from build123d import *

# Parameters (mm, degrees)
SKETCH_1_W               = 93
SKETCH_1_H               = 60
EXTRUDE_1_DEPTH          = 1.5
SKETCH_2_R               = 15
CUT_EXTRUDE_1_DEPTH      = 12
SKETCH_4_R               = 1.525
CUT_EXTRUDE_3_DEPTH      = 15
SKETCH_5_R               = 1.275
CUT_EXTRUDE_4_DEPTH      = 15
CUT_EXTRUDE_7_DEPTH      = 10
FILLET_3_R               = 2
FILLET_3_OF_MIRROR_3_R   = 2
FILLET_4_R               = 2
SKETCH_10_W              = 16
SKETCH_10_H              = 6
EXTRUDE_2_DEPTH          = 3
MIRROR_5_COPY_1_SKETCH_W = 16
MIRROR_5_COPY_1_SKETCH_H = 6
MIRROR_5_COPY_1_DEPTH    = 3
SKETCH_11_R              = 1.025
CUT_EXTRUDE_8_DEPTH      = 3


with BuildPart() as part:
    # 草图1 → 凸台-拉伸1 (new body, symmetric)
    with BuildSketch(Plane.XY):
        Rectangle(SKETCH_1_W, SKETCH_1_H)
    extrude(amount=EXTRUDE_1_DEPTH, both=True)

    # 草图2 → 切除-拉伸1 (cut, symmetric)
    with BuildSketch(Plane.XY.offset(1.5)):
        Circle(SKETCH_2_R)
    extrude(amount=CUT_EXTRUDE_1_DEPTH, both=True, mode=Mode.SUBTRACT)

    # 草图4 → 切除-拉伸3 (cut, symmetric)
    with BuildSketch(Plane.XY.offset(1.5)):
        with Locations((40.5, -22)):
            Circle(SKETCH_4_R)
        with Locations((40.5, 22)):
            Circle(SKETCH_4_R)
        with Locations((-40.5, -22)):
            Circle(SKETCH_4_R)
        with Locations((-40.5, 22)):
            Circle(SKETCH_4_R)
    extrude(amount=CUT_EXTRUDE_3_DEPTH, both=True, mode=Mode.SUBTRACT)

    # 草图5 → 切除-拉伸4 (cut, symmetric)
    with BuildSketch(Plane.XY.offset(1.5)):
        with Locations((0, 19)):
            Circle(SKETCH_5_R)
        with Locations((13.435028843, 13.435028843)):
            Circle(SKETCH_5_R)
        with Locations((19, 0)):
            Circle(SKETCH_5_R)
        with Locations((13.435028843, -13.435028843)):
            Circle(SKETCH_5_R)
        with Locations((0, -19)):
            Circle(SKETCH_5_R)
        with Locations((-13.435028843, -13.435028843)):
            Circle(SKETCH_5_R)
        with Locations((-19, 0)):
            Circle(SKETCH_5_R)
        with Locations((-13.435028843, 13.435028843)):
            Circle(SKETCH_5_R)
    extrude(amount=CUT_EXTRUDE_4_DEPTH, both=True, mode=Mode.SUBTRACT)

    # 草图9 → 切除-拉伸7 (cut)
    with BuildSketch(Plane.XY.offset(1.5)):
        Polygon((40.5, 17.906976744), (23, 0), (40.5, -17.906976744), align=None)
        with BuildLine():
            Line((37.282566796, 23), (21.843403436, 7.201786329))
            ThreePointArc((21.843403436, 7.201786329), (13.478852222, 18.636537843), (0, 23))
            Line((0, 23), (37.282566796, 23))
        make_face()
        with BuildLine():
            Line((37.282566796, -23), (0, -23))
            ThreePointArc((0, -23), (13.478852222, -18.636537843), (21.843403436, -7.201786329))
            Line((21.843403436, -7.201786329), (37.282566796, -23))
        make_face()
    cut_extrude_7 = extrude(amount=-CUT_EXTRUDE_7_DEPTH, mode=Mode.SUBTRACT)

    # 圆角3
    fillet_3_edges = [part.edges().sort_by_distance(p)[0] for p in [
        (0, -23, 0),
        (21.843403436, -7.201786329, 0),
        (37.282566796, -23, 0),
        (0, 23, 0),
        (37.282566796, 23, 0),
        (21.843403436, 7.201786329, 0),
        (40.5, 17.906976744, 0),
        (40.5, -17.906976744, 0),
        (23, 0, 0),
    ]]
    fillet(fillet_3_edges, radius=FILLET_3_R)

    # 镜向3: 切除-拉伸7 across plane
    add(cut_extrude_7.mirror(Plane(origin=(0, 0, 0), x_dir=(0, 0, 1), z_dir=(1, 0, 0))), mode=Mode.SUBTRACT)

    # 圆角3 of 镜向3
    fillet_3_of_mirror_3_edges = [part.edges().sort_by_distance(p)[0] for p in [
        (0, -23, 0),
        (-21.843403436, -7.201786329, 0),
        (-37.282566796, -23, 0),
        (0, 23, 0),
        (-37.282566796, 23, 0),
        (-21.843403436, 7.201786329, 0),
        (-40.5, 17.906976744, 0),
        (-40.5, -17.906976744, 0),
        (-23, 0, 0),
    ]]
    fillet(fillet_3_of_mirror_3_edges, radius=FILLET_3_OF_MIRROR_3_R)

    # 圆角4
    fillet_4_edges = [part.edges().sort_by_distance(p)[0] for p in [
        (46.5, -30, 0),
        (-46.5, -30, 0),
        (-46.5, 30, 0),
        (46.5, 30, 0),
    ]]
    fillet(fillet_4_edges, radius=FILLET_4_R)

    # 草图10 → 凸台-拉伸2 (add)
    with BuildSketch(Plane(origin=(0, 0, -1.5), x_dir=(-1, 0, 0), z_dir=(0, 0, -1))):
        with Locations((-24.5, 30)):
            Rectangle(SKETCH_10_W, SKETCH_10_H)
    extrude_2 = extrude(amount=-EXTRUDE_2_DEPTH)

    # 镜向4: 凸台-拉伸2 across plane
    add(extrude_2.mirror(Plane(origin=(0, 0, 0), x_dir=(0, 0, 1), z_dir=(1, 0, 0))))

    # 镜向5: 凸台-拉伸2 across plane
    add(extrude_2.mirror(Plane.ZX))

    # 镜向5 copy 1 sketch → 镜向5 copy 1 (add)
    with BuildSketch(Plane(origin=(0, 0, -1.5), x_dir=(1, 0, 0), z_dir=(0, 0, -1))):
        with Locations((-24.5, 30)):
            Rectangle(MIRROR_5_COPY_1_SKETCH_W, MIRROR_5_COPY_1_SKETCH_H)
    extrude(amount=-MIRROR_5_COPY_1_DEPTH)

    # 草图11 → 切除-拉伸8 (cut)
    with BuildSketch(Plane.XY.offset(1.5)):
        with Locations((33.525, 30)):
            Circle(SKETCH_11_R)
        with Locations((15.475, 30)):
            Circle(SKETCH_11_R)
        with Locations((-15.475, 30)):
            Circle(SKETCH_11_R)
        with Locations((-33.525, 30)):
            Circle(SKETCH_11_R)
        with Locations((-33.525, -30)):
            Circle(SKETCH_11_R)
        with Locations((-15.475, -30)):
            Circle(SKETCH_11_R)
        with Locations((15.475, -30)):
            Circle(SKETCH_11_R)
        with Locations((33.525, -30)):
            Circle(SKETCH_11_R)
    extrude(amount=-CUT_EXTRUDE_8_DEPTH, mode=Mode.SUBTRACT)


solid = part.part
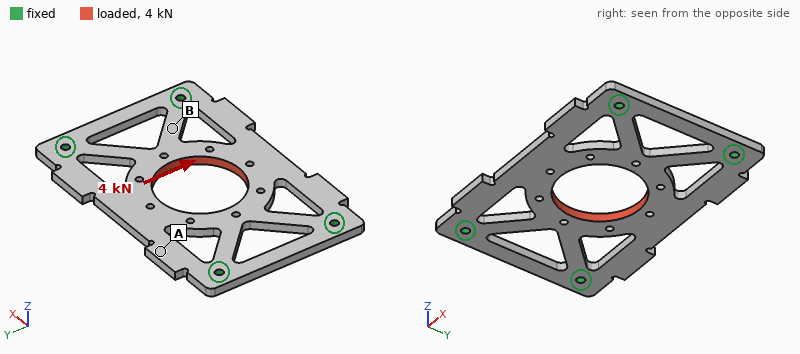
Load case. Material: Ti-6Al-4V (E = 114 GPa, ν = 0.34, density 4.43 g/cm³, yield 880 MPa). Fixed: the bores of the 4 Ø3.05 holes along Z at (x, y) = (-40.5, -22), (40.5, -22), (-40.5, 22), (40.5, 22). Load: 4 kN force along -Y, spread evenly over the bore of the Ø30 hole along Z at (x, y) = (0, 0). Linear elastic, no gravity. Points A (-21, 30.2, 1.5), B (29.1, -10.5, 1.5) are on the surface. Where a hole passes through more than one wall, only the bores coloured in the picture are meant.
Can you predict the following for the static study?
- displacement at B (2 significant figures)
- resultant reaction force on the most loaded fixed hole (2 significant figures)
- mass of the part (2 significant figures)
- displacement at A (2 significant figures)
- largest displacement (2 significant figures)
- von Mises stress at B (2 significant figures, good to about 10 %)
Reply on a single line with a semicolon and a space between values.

15 µm; 1.3 kN; 48 g; 23 µm; 36 µm; 69 MPa
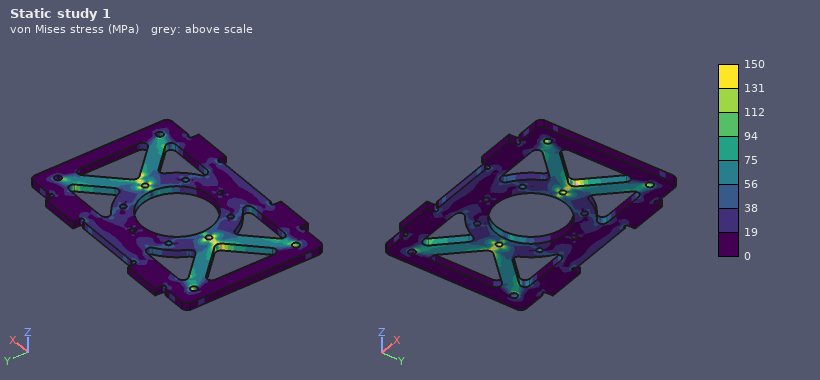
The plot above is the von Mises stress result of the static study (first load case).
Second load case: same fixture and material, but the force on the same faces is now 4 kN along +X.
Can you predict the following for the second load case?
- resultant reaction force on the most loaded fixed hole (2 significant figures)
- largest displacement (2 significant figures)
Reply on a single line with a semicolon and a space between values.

1.1 kN; 18 µm
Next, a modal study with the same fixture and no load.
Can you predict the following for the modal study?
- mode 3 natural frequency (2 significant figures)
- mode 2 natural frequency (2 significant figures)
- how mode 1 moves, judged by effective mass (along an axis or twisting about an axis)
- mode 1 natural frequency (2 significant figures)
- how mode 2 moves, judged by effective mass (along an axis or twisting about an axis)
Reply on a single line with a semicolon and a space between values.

4500 Hz; 2500 Hz; along Z; 2000 Hz; twisting about X
